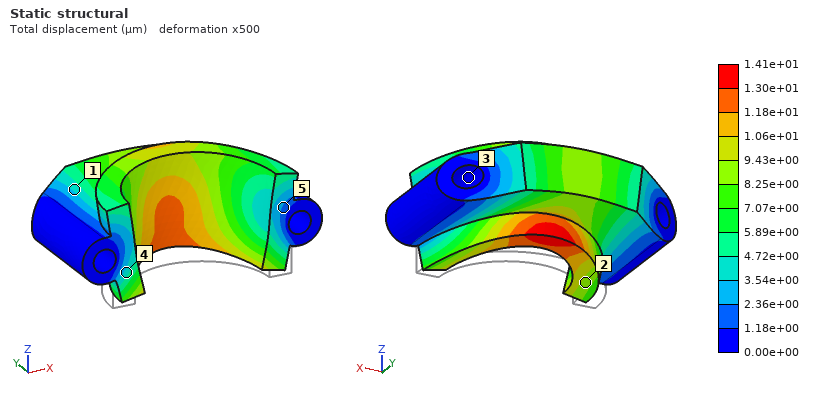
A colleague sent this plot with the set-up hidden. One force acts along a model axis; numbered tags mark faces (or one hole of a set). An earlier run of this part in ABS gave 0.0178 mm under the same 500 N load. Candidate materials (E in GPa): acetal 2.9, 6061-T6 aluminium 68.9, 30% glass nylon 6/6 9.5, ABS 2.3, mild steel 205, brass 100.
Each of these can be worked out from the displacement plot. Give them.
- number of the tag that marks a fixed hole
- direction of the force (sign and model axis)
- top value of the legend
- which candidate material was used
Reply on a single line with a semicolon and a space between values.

3; +Z; 1.41e+01 µm; acetal
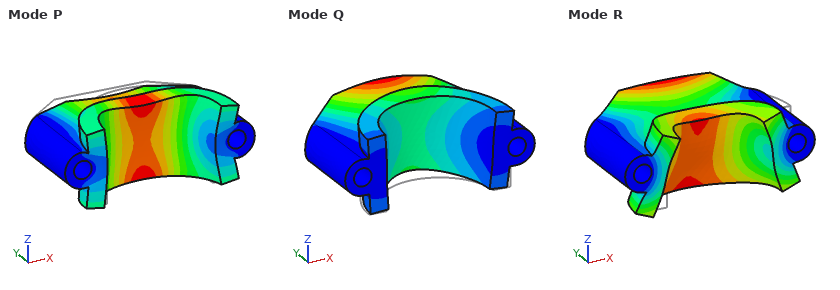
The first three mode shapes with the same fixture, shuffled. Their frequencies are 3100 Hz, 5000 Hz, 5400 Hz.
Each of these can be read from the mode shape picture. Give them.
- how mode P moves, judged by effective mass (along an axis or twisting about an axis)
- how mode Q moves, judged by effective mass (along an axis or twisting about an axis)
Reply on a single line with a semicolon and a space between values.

along Y; along Z
